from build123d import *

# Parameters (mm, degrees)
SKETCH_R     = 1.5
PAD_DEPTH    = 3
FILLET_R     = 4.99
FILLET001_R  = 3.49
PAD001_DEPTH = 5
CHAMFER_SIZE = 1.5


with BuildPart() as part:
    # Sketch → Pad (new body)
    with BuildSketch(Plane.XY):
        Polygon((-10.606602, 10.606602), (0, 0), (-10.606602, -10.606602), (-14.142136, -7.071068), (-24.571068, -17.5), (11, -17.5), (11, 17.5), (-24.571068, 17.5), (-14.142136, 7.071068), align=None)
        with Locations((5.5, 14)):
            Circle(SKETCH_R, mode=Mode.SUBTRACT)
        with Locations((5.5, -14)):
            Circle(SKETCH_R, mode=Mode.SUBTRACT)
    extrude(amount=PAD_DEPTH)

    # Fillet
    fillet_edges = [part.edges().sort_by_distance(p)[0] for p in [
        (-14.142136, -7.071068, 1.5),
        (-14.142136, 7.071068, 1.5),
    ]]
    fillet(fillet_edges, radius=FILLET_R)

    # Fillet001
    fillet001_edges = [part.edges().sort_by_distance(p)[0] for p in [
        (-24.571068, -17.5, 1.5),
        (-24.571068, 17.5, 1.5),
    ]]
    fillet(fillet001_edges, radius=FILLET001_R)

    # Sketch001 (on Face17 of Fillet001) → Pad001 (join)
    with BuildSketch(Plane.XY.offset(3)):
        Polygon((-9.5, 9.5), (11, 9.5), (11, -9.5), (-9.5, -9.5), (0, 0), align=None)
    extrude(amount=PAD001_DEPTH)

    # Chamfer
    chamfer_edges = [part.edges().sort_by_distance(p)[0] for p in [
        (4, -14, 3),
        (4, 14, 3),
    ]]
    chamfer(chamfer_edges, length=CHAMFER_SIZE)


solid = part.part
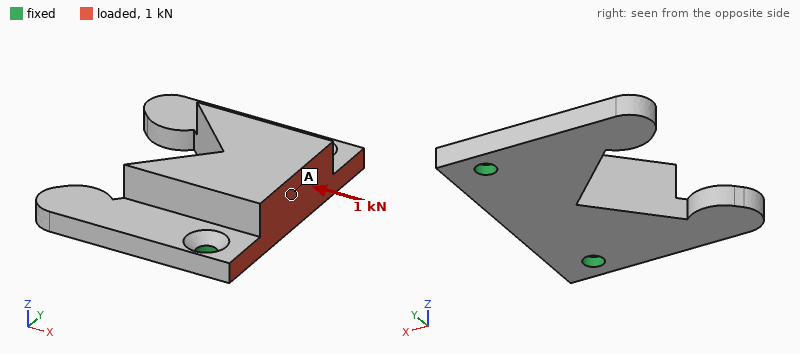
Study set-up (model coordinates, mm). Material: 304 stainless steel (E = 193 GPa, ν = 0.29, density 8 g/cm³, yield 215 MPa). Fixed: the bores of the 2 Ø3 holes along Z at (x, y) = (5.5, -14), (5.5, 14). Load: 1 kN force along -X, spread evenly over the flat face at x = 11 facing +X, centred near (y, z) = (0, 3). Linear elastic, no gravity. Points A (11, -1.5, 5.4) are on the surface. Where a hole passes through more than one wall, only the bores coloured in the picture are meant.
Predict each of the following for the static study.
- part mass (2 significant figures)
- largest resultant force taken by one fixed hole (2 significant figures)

30 g
500 N
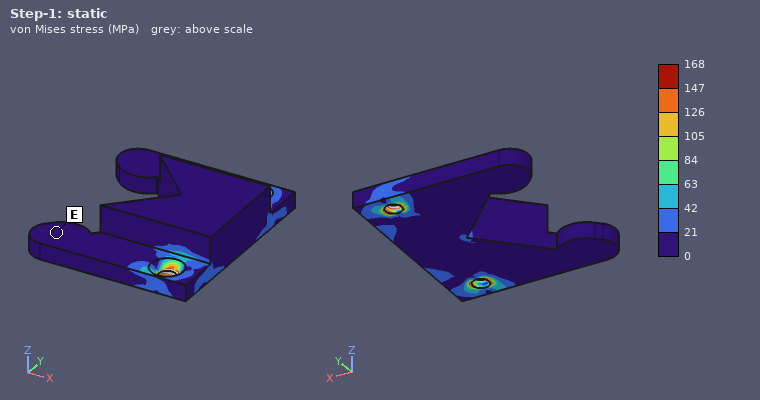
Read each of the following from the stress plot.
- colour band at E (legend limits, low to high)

0 to 21 MPa
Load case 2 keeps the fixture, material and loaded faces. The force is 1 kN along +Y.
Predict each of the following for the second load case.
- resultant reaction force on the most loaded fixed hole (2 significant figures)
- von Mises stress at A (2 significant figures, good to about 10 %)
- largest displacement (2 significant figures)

540 N
12 MPa
1.7 µm
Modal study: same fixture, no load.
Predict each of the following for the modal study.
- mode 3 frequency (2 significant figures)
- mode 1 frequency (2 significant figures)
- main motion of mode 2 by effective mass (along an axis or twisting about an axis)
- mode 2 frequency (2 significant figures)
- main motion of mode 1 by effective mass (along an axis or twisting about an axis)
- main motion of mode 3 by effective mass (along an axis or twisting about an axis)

14 kHz
4200 Hz
twisting about X
8300 Hz
along Z
along X
